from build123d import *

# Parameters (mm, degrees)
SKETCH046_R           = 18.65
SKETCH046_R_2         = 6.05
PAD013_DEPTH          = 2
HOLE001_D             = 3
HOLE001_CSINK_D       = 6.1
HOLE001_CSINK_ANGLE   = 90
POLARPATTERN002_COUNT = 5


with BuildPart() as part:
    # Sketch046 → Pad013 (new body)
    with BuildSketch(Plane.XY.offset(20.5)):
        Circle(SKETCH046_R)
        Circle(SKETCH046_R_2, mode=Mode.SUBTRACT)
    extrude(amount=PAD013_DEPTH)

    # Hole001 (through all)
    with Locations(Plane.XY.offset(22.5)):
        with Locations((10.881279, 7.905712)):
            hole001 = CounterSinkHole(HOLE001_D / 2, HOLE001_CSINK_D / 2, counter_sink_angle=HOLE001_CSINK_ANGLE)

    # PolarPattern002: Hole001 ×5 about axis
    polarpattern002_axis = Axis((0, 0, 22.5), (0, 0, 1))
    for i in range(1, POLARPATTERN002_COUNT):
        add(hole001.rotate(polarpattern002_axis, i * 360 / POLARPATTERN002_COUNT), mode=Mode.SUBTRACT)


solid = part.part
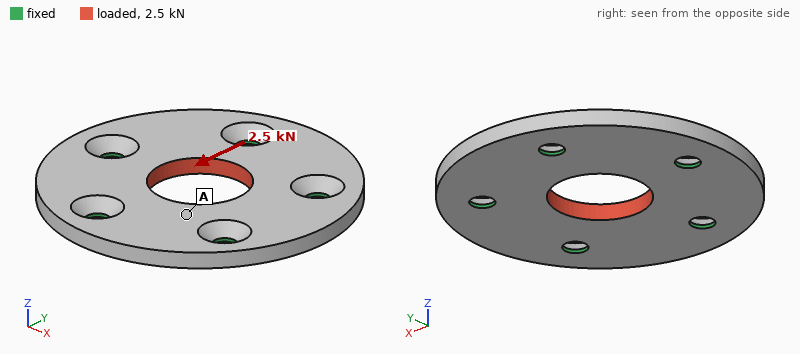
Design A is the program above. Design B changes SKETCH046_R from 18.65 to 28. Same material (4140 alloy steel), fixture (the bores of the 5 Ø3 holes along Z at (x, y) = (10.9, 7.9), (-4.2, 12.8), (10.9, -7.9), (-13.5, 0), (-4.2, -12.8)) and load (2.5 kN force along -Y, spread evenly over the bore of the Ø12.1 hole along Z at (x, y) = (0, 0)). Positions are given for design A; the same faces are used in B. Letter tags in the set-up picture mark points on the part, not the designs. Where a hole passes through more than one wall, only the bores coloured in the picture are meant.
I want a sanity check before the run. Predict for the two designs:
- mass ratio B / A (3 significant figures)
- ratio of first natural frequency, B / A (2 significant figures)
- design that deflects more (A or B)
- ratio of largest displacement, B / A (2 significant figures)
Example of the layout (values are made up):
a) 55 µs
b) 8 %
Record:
a) 2.52
b) 0.28
c) B
d) 1.6
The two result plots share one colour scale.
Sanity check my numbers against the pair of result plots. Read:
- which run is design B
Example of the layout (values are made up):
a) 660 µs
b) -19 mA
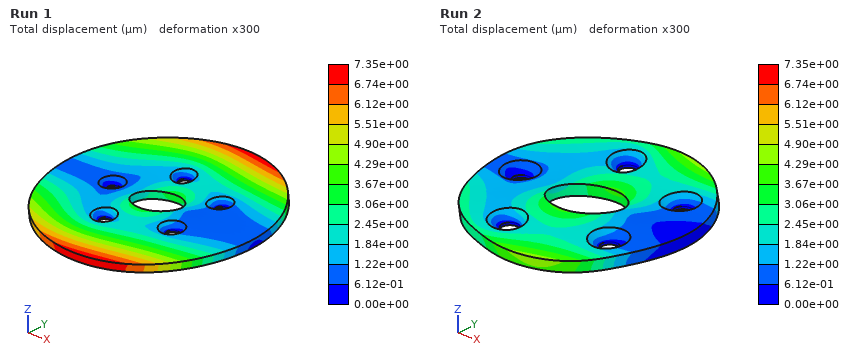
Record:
a) Run 1
